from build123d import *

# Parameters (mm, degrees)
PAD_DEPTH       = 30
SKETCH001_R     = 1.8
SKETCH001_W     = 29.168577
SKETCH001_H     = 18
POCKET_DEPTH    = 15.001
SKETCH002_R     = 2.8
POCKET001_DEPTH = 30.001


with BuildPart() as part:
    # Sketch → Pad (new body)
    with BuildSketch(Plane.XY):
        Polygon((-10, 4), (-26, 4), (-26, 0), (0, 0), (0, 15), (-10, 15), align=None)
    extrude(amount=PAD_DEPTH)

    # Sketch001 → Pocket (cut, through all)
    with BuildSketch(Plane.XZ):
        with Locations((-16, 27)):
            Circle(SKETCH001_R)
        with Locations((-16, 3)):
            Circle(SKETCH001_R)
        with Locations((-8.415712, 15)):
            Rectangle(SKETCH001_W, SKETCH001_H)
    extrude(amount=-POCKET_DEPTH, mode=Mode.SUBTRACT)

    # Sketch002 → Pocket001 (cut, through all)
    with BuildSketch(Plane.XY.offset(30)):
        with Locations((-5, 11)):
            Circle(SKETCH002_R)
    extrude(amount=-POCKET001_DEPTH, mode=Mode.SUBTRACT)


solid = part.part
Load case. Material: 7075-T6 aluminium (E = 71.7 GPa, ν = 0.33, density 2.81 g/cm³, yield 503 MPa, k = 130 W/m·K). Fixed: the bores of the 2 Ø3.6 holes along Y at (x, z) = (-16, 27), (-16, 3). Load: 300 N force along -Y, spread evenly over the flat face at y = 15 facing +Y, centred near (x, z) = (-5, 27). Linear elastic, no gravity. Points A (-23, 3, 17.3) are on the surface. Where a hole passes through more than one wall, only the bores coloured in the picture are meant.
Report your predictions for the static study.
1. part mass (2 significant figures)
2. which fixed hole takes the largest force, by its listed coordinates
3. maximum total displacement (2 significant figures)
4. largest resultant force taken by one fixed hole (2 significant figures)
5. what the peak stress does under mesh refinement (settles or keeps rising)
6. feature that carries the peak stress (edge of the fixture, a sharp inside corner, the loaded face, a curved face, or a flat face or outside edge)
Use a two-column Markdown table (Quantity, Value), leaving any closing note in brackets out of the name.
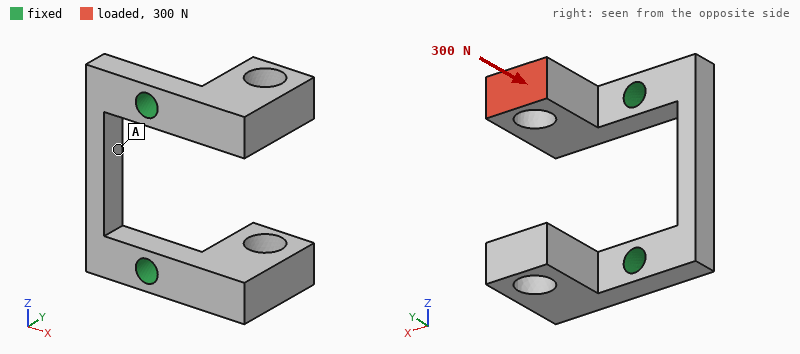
| Quantity | Value |
|---|---|
| part mass | 6.8 g |
| which fixed hole takes the largest force, by its listed coordinates | (-16, 27) |
| maximum total displacement | 0.10 mm |
| largest resultant force taken by one fixed hole | 300 N |
| what the peak stress does under mesh refinement | keeps rising |
| feature that carries the peak stress | edge of the fixture |
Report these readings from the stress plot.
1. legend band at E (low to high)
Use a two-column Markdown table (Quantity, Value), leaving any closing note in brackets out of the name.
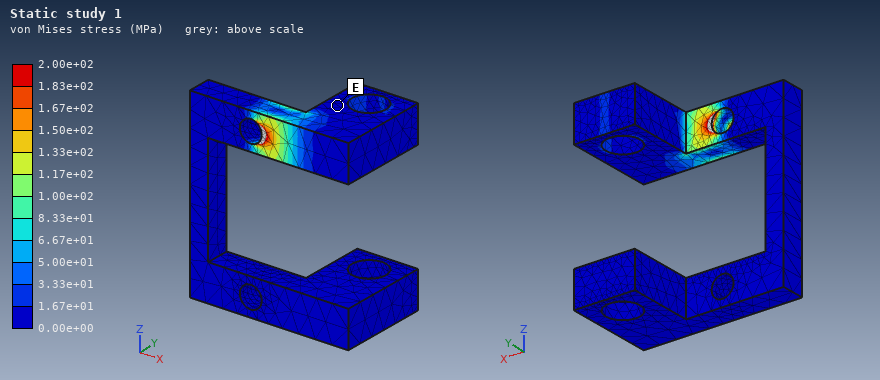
| Quantity | Value |
|---|---|
| legend band at E | 0.00e+00 to 1.67e+01 MPa |
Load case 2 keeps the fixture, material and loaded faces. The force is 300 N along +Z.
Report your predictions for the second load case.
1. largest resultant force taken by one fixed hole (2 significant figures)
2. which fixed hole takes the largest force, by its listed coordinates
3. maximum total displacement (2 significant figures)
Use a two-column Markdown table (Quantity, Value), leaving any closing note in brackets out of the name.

| Quantity | Value |
|---|---|
| largest resultant force taken by one fixed hole | 310 N |
| which fixed hole takes the largest force, by its listed coordinates | (-16, 27) |
| maximum total displacement | 0.21 mm |
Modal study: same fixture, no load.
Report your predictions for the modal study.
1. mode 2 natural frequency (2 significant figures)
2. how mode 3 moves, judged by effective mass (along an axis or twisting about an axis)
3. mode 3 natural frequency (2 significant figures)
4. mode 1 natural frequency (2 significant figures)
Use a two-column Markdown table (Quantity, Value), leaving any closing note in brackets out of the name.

| Quantity | Value |
|---|---|
| mode 2 natural frequency | 6400 Hz |
| how mode 3 moves, judged by effective mass | along Z |
| mode 3 natural frequency | 7800 Hz |
| mode 1 natural frequency | 6400 Hz |
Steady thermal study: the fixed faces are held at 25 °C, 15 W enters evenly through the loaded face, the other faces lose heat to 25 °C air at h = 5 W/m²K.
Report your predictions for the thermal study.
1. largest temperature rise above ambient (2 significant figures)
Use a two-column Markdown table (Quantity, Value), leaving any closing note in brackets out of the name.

| Quantity | Value |
|---|---|
| largest temperature rise above ambient | 72 K |
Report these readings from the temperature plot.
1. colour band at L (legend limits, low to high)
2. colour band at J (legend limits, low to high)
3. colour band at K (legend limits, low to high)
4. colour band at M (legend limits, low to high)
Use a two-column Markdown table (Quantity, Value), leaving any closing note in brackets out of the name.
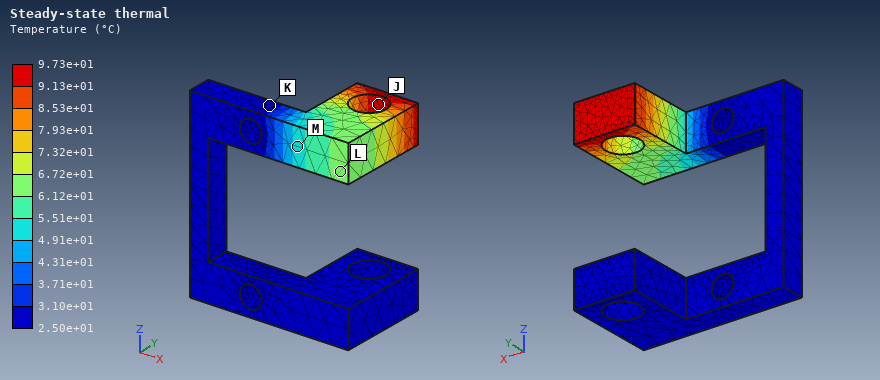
| Quantity | Value |
|---|---|
| colour band at L | 6.12e+01 to 6.72e+01 °C |
| colour band at J | 9.13e+01 to 9.73e+01 °C |
| colour band at K | 2.50e+01 to 3.10e+01 °C |
| colour band at M | 4.91e+01 to 5.51e+01 °C |
